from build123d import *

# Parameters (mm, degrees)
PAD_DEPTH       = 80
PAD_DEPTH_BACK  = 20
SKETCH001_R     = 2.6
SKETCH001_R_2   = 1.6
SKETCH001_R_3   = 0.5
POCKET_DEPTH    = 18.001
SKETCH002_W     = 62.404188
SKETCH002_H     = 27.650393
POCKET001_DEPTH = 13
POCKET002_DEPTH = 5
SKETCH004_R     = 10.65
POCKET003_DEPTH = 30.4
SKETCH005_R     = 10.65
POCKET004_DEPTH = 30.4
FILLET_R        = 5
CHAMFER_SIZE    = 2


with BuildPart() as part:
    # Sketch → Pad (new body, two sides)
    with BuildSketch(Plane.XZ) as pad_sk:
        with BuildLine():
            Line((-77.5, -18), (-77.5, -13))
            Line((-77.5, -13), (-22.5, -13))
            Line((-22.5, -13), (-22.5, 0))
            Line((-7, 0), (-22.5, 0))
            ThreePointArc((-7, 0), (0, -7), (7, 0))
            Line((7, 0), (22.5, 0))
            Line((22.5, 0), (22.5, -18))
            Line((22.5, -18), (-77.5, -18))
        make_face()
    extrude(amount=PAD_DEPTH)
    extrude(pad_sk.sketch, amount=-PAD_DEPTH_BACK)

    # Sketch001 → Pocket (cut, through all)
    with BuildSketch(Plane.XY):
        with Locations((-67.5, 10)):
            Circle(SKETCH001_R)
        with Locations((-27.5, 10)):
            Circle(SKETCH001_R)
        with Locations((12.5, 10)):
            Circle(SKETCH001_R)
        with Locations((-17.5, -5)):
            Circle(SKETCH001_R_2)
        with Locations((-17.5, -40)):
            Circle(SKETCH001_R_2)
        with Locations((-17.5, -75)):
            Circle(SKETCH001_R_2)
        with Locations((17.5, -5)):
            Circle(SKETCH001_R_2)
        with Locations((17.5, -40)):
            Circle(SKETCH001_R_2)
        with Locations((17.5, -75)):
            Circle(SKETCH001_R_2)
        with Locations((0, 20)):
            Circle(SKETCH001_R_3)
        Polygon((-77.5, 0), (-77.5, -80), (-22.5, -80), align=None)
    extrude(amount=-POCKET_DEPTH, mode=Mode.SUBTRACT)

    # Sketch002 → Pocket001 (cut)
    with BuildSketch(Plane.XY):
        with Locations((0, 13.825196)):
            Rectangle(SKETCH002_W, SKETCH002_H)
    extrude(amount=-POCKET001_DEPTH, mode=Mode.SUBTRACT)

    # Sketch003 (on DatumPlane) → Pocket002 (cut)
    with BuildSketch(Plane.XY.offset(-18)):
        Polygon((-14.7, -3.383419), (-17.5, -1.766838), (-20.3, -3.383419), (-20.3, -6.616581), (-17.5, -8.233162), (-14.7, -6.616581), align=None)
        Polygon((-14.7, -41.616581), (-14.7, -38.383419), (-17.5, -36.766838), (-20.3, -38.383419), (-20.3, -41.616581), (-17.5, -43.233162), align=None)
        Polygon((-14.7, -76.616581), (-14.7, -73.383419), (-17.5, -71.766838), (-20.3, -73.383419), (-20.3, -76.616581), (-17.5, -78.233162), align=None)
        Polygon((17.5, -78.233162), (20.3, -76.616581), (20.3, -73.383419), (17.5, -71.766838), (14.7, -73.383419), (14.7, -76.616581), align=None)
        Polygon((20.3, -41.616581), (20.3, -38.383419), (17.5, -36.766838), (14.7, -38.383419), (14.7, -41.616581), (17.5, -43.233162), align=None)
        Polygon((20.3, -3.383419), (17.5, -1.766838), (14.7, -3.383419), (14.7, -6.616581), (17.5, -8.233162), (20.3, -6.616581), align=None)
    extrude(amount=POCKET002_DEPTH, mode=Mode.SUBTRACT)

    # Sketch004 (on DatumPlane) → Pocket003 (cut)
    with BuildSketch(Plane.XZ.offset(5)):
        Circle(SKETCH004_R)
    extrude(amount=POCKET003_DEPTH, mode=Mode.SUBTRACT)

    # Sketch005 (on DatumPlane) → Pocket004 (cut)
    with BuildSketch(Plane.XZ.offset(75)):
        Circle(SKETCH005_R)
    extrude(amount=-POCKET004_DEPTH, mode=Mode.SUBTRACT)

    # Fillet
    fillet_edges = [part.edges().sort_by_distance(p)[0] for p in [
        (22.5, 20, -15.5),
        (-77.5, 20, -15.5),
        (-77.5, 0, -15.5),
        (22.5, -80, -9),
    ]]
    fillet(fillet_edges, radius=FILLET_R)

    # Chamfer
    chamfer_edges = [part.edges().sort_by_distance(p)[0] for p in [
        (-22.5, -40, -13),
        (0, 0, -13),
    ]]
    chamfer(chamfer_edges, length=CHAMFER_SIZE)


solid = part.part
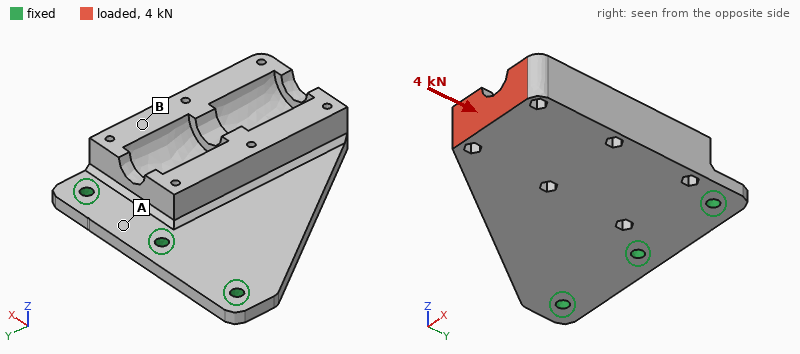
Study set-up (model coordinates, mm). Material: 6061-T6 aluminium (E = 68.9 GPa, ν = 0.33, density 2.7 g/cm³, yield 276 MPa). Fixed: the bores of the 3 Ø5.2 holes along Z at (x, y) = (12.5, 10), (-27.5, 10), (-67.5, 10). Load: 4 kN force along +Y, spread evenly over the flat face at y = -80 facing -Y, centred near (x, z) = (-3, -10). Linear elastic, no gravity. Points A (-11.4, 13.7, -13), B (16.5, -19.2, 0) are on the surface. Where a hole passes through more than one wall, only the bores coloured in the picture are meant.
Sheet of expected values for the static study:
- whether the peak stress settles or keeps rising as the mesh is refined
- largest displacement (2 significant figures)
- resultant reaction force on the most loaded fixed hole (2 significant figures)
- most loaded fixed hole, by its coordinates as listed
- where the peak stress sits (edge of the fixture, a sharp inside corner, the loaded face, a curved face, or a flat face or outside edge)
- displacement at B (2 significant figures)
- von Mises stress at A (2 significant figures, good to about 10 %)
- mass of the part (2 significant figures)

keeps rising
0.49 mm
2.5 kN
(12.5, 10)
edge of the fixture
0.17 mm
21 MPa
190 g
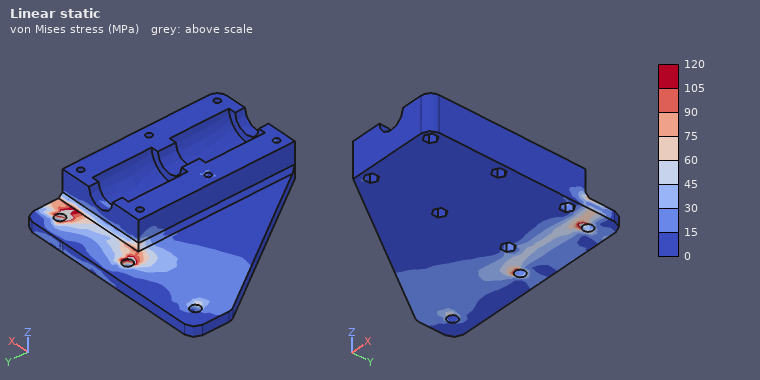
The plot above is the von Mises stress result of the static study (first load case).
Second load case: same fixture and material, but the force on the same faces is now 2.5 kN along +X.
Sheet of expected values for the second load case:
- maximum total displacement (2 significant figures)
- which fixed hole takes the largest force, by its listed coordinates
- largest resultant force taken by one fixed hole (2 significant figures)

98 µm
(12.5, 10)
3.4 kN
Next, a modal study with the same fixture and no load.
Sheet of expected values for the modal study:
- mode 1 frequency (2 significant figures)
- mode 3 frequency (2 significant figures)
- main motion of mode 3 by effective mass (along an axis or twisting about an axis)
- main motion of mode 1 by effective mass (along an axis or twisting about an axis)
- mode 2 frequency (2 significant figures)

510 Hz
4600 Hz
along X
along Z
2800 Hz
